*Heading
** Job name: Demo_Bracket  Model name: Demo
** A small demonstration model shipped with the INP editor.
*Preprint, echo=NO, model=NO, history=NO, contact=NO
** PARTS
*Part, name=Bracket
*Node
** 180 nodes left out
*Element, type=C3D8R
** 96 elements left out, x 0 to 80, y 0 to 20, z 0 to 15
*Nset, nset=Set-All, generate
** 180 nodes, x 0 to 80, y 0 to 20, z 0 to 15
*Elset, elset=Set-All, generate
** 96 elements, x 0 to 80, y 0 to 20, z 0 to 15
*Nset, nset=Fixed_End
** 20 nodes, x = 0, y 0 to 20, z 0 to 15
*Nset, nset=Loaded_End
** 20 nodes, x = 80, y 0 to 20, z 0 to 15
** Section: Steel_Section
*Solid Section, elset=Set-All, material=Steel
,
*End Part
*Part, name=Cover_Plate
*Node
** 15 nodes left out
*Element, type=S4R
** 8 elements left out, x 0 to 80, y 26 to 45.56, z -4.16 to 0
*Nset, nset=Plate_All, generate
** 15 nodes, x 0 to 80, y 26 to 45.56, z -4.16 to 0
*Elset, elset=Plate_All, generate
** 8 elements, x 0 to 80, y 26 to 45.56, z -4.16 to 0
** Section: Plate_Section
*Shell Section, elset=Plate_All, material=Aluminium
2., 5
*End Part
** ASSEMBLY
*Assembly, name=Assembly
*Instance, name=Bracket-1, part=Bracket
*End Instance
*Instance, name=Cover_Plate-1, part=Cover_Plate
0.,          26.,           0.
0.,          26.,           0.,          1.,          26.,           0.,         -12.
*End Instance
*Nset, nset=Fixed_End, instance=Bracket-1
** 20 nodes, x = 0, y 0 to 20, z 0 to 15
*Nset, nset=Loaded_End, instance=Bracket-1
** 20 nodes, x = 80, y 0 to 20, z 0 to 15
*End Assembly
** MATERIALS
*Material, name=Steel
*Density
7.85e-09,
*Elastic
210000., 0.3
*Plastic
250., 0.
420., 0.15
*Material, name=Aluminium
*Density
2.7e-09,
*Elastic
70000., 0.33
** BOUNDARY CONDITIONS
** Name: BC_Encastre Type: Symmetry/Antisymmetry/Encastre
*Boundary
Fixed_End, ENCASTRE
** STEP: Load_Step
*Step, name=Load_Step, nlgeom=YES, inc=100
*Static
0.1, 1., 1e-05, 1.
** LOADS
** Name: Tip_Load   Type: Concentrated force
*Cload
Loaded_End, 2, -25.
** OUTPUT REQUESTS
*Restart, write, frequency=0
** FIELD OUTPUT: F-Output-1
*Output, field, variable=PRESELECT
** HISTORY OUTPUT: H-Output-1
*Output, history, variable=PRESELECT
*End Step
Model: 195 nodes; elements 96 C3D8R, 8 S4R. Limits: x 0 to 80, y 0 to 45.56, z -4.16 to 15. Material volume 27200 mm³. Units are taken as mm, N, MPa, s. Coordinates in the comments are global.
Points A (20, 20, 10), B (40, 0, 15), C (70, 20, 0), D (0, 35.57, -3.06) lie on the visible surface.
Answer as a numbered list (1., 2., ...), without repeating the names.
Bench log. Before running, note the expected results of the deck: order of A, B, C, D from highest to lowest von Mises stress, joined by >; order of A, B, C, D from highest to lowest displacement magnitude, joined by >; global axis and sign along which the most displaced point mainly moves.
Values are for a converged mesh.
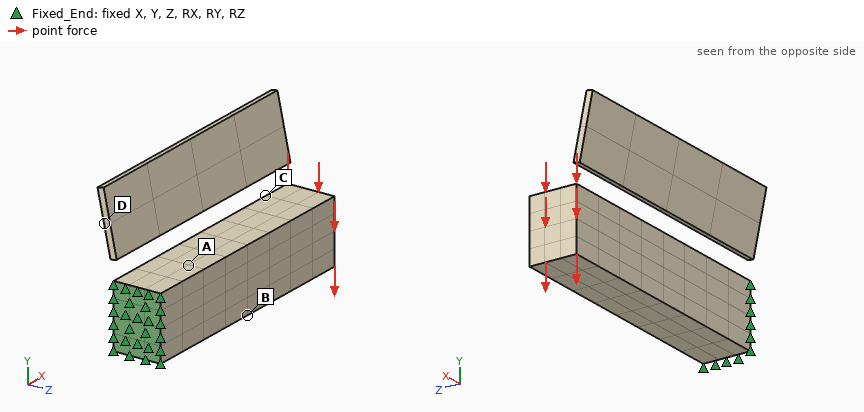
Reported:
1. A > B > C > D
2. C > B > A > D
3. -Y
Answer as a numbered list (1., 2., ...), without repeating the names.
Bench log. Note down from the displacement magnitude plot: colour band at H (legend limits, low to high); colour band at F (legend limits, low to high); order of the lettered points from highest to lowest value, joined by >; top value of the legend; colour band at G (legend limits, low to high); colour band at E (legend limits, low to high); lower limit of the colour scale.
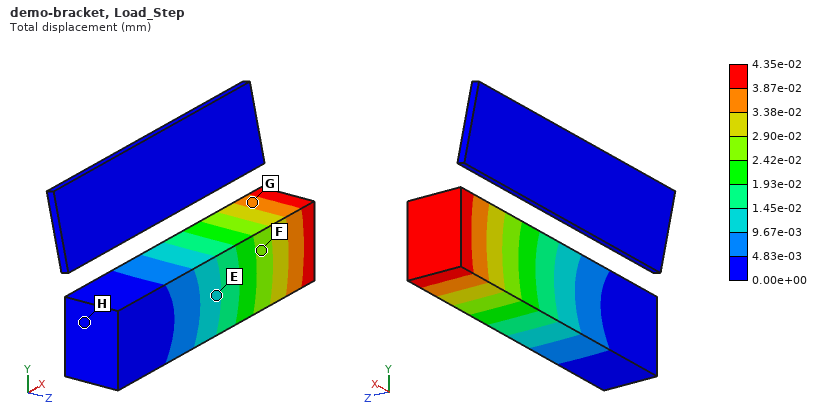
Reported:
1. 0.00e+00 to 4.83e-03 mm
2. 2.42e-02 to 2.90e-02 mm
3. G > F > E > H
4. 4.35e-02 mm
5. 3.38e-02 to 3.87e-02 mm
6. 9.67e-03 to 1.45e-02 mm
7. 0.00e+00 mm
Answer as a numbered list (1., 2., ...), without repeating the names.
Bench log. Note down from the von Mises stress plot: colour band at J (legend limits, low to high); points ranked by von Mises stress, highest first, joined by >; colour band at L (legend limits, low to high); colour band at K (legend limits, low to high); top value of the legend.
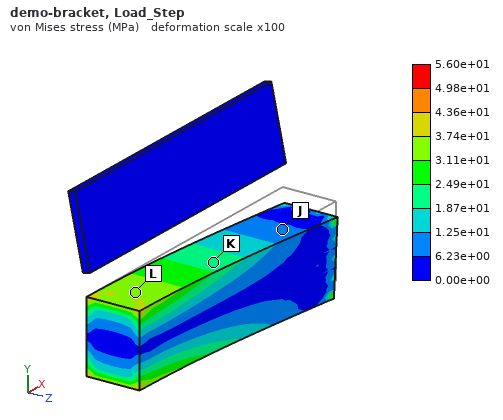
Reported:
1. 6.23e+00 to 1.25e+01 MPa
2. L > K > J
3. 3.11e+01 to 3.74e+01 MPa
4. 1.87e+01 to 2.49e+01 MPa
5. 5.60e+01 MPa
